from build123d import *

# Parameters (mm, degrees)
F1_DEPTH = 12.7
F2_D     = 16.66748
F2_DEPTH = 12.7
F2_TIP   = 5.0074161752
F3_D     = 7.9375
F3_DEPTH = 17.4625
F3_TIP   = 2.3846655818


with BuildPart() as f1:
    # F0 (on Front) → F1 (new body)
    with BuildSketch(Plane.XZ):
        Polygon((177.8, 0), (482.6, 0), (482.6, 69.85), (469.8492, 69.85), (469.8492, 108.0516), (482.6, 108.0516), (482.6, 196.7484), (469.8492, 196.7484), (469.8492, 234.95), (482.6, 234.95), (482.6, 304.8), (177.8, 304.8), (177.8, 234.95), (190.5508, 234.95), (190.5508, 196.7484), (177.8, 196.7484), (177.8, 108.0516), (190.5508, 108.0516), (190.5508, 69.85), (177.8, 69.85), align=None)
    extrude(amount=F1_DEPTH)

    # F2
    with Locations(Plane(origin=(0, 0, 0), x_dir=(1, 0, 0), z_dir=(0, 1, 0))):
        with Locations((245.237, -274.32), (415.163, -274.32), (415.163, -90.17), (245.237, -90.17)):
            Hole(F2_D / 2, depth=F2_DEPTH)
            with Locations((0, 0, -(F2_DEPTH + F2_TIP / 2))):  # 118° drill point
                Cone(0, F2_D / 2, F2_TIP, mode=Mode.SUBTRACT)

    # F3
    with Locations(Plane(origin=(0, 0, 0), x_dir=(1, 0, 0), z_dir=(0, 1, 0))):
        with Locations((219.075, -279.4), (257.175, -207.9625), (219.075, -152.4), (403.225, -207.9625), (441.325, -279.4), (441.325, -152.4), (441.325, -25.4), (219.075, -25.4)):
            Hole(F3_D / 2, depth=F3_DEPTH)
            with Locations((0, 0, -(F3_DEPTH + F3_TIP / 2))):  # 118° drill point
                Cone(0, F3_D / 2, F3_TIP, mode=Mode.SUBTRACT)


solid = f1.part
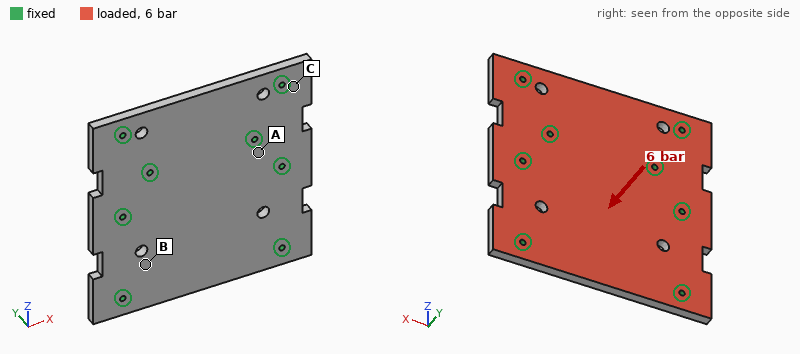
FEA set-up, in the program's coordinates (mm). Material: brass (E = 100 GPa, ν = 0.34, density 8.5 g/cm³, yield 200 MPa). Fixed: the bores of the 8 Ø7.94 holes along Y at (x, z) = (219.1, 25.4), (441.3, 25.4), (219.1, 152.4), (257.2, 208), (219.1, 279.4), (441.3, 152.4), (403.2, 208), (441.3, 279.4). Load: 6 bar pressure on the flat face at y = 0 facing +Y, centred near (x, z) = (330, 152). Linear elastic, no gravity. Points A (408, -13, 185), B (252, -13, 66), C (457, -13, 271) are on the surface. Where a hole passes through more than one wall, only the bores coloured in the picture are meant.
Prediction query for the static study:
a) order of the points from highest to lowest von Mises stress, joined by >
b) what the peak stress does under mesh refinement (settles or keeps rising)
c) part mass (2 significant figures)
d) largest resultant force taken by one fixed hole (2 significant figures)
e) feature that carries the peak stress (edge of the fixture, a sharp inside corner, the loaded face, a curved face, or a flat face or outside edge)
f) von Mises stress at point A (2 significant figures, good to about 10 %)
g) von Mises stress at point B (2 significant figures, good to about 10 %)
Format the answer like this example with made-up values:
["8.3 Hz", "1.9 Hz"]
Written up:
["A > B > C", "keeps rising", "9.7 kg", "8.5 kN", "edge of the fixture", "37 MPa", "22 MPa"]
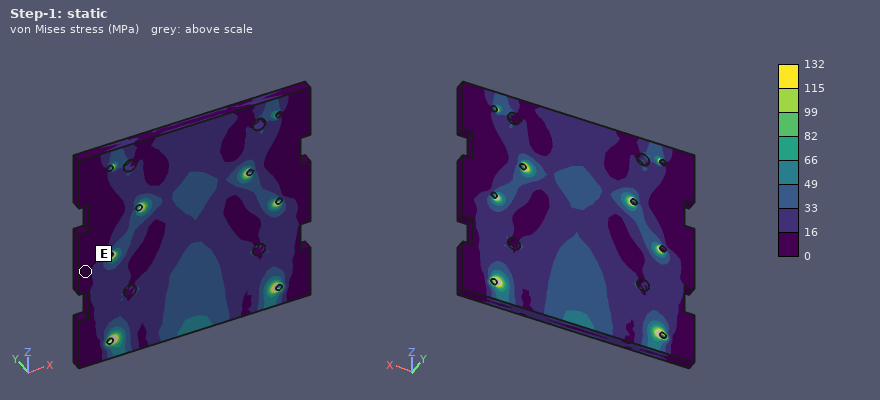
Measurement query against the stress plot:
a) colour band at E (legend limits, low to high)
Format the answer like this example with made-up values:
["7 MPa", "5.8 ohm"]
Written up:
["0 to 16 MPa"]
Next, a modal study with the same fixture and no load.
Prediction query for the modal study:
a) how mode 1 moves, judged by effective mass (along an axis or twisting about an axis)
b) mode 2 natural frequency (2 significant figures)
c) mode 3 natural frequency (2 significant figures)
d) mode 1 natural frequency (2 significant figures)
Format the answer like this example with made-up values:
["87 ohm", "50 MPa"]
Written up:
["along Y", "1100 Hz", "1400 Hz", "820 Hz"]
